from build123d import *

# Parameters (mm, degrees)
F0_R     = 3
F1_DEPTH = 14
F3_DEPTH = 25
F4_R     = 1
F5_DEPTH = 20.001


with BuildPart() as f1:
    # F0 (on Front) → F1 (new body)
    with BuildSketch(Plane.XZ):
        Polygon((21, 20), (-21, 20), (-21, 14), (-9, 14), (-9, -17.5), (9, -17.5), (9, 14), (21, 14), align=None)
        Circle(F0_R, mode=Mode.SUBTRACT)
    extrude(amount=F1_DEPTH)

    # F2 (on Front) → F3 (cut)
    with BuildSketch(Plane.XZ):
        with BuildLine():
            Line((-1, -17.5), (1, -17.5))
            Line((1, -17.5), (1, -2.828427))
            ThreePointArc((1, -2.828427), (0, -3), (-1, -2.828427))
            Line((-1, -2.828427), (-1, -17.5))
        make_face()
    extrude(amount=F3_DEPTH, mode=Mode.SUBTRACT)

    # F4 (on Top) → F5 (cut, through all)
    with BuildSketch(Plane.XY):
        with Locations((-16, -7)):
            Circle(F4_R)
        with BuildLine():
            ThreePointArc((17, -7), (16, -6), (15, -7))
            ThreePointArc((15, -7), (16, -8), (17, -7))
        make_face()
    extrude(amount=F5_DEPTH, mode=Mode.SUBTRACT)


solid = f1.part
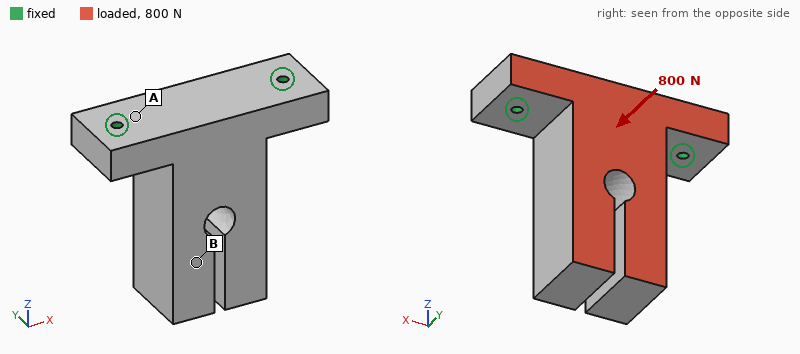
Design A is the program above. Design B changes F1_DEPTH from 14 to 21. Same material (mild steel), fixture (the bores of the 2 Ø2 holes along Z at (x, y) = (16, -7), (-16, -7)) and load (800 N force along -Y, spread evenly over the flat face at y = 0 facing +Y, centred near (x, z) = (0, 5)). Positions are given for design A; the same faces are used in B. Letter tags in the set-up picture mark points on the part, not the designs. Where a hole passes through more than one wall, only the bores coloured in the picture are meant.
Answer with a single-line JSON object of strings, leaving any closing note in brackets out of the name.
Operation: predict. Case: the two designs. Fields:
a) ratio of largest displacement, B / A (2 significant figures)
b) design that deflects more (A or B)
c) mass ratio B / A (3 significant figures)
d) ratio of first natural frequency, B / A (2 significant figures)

{"ratio of largest displacement, B / A": "0.76", "design that deflects more": "A", "mass ratio B / A": "1.50", "ratio of first natural frequency, B / A": "0.92"}
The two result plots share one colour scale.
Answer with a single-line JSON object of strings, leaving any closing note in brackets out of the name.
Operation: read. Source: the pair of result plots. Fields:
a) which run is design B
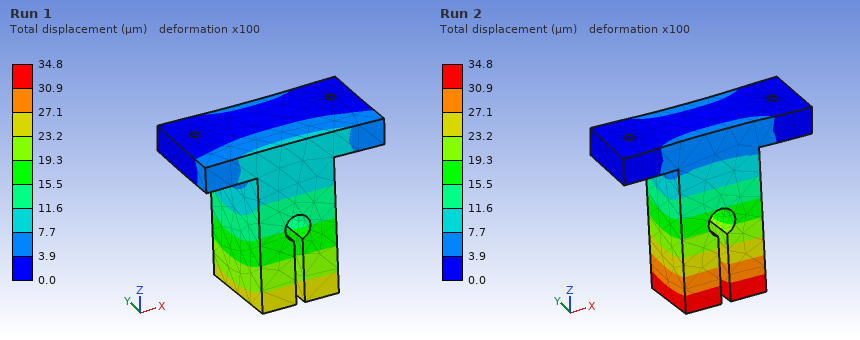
{"which run is design B": "Run 1"}
